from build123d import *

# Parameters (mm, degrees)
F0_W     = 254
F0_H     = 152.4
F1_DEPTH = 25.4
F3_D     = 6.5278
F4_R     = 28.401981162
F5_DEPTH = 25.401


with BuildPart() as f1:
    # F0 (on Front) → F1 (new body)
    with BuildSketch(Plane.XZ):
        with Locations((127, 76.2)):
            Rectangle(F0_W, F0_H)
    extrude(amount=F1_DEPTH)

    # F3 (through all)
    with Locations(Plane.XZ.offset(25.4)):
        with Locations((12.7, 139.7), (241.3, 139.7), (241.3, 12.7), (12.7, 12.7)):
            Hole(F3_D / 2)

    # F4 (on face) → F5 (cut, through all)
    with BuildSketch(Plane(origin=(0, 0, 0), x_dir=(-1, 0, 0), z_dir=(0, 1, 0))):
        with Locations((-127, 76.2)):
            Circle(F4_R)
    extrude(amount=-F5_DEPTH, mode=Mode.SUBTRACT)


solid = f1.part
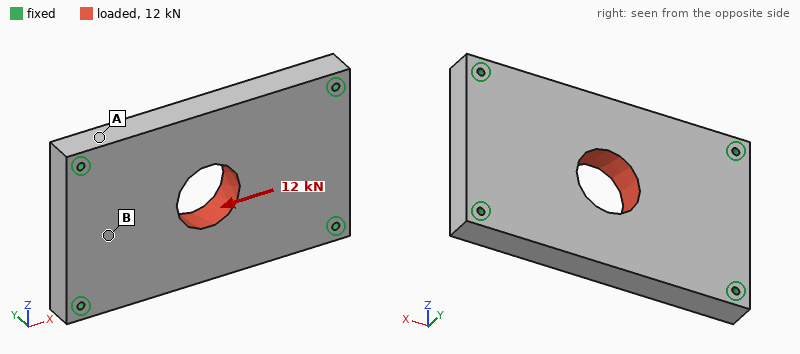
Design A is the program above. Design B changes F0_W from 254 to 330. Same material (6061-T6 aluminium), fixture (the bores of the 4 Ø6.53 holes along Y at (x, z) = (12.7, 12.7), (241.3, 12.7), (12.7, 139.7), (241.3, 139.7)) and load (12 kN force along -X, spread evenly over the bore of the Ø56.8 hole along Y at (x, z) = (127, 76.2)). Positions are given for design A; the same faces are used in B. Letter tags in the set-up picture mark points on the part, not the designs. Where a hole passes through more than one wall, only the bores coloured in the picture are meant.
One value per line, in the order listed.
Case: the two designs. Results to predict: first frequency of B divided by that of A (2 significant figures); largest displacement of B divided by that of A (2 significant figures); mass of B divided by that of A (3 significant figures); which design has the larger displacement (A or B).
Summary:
1.0
0.90
1.32
A
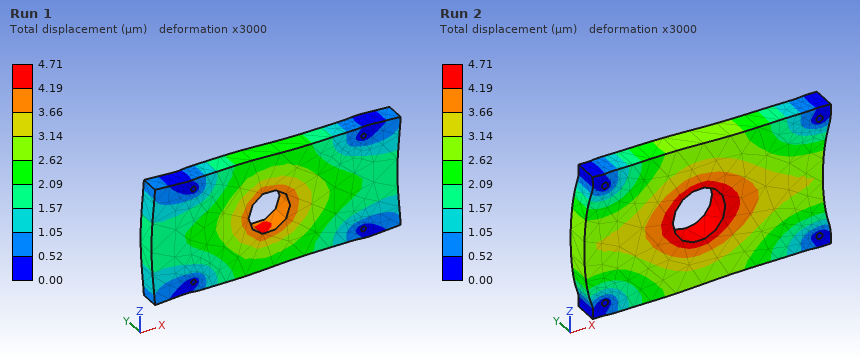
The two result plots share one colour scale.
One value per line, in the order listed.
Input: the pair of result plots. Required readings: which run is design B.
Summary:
Run 1
